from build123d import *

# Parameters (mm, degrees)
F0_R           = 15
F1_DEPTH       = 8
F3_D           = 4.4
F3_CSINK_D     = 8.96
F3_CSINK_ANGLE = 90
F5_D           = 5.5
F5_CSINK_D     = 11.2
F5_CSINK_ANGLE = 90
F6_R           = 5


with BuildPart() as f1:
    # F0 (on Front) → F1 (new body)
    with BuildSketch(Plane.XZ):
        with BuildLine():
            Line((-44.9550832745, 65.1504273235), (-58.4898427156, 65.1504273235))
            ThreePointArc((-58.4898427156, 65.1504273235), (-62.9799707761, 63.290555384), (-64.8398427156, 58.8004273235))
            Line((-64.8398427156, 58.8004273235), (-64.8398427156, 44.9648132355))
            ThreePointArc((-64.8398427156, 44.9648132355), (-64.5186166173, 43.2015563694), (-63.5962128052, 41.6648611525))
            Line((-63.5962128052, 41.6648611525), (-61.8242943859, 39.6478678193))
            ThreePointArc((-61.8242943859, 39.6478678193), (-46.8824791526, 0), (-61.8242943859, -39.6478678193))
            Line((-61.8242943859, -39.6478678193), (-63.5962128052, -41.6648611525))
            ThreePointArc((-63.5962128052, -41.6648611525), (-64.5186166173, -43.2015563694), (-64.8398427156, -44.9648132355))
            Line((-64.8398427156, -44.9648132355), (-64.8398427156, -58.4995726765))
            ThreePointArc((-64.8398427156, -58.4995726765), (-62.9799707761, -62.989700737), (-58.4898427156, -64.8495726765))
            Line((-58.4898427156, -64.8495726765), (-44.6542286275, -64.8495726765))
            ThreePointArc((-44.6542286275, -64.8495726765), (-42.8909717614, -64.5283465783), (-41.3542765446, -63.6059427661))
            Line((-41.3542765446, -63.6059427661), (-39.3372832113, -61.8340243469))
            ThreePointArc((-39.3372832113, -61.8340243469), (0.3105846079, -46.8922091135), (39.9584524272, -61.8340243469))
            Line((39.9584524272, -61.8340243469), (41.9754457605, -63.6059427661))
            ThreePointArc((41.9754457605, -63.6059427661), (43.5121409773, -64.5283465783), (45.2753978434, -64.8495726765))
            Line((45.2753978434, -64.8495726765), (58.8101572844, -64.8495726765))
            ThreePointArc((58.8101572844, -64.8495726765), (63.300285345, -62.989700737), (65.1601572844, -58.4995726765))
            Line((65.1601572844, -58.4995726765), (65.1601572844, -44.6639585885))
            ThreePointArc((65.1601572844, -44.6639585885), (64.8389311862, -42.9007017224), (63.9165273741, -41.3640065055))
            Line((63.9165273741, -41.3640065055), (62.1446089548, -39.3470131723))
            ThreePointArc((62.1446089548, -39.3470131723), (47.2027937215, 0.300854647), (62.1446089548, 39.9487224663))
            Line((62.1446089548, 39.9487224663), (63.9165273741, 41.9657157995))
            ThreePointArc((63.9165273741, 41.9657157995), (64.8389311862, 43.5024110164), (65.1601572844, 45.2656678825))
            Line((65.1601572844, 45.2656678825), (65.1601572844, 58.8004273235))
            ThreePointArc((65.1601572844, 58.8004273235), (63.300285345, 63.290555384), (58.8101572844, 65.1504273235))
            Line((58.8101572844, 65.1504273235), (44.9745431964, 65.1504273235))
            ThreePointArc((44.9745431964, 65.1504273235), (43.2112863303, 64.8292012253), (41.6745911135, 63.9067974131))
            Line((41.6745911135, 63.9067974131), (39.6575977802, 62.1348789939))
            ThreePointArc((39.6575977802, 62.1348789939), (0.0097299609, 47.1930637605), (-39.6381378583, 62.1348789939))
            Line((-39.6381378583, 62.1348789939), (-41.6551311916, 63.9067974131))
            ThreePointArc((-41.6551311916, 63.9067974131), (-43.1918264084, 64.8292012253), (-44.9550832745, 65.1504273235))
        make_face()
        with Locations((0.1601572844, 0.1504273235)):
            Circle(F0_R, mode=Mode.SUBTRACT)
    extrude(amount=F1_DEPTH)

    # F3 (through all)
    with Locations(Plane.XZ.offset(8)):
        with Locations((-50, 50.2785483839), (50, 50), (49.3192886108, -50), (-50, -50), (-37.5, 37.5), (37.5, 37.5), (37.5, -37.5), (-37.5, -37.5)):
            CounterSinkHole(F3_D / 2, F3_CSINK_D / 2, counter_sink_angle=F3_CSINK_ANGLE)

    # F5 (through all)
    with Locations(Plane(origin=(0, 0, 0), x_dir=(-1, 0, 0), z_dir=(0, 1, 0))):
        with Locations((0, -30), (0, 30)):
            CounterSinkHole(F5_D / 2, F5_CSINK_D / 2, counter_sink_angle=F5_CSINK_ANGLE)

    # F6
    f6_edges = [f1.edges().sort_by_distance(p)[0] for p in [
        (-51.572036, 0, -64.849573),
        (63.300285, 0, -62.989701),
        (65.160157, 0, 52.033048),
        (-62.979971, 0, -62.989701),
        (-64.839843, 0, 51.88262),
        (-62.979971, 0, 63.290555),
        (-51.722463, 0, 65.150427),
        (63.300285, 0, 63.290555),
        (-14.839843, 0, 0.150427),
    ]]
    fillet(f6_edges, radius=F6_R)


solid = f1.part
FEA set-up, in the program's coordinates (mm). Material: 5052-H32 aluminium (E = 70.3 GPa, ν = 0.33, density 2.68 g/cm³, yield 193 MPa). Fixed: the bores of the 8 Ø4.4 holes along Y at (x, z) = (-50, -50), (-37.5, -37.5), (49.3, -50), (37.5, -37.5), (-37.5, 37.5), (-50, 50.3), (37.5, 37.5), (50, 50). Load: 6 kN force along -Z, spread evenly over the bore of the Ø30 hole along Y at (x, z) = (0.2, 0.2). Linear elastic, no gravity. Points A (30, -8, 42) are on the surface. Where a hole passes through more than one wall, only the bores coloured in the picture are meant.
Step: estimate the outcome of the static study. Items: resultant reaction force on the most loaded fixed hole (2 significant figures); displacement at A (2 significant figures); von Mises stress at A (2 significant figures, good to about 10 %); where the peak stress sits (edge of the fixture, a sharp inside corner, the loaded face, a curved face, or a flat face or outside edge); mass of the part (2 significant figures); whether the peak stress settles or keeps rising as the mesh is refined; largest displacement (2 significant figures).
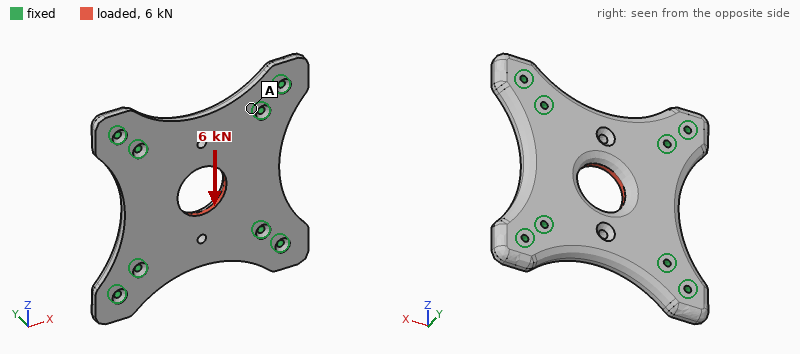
1.3 kN
1.9 µm
5.1 MPa
edge of the fixture
240 g
keeps rising
9.5 µm
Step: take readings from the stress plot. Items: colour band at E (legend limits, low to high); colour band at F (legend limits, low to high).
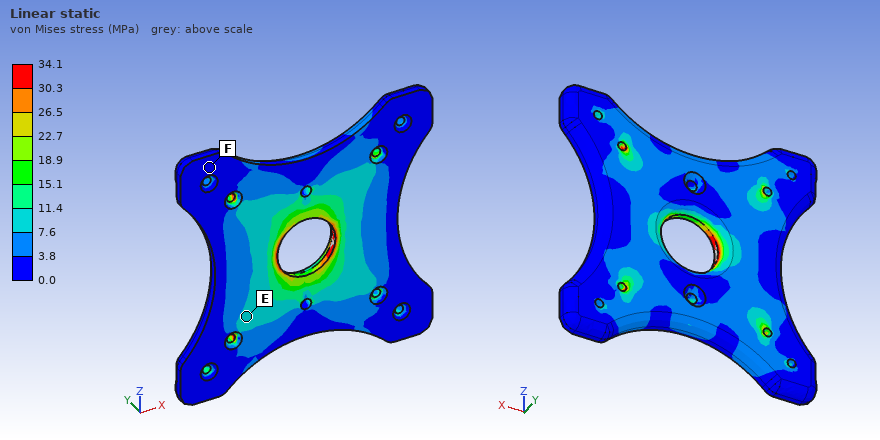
7.6 to 11.4 MPa
0.0 to 3.8 MPa
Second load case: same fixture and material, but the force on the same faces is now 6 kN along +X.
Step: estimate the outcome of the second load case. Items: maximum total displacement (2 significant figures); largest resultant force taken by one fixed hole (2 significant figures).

9.5 µm
1.3 kN
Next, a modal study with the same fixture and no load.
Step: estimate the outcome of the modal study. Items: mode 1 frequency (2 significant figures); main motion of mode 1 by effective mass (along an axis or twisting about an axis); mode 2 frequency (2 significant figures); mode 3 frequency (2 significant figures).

4600 Hz
along Y
6900 Hz
6900 Hz
